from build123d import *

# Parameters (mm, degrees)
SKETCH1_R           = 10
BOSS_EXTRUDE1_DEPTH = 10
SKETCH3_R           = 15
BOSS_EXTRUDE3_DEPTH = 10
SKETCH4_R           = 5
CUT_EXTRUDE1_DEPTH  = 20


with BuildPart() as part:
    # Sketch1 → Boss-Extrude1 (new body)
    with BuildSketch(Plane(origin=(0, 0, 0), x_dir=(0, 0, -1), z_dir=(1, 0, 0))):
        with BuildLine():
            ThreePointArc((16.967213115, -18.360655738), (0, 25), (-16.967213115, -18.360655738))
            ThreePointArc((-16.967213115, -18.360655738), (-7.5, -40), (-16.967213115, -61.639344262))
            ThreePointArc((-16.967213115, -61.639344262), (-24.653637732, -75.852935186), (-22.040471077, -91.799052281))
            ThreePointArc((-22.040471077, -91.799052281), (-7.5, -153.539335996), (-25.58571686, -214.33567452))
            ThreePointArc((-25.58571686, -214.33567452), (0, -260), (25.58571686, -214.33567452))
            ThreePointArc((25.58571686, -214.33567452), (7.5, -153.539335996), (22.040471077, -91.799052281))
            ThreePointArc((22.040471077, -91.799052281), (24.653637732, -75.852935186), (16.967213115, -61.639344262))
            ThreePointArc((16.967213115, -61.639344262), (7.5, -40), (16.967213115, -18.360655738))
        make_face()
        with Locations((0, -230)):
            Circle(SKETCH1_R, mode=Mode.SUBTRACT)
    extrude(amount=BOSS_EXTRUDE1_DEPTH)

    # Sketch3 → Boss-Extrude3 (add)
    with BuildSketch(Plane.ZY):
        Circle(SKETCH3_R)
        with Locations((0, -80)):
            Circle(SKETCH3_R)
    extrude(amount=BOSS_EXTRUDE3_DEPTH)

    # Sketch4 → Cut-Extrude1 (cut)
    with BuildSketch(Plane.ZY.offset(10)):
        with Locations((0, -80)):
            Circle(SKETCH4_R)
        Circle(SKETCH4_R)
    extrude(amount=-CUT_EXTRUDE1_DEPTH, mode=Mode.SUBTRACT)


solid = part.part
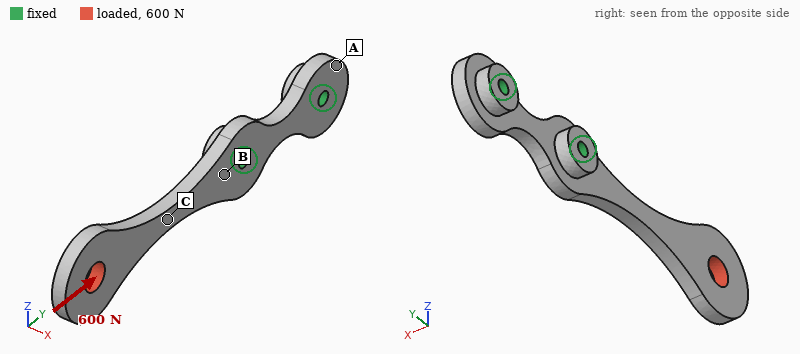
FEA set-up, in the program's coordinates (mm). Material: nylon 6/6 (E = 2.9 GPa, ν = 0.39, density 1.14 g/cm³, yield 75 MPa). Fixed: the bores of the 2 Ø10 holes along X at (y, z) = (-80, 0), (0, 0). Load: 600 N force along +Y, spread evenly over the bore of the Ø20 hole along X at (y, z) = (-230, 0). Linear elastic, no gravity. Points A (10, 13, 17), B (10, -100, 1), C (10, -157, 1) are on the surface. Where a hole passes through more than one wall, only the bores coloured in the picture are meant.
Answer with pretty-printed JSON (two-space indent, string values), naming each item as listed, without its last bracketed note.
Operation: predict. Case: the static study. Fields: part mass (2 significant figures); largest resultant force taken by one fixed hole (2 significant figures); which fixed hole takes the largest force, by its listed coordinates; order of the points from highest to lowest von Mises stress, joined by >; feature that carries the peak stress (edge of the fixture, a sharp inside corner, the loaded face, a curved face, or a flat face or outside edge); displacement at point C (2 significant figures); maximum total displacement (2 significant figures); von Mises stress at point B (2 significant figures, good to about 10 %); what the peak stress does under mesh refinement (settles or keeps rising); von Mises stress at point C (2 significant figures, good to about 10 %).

{
  "part mass": "120 g",
  "largest resultant force taken by one fixed hole": "580 N",
  "which fixed hole takes the largest force, by its listed coordinates": "(-80, 0)",
  "order of the points from highest to lowest von Mises stress, joined by >": "C > B > A",
  "feature that carries the peak stress": "edge of the fixture",
  "displacement at point C": "0.084 mm",
  "maximum total displacement": "0.17 mm",
  "von Mises stress at point B": "2.4 MPa",
  "what the peak stress does under mesh refinement": "keeps rising",
  "von Mises stress at point C": "3.8 MPa"
}
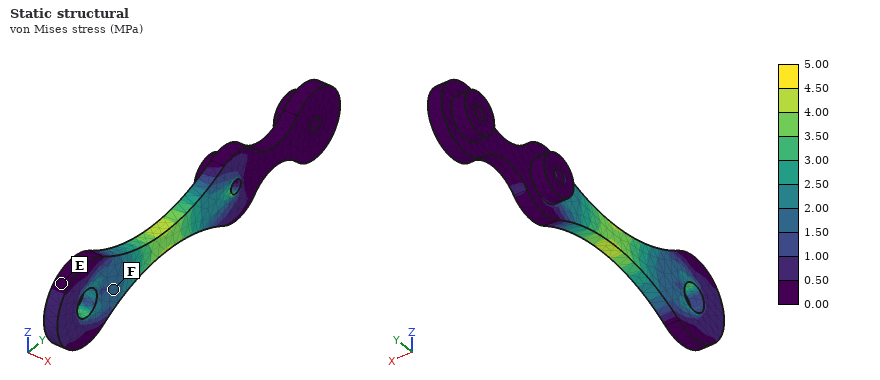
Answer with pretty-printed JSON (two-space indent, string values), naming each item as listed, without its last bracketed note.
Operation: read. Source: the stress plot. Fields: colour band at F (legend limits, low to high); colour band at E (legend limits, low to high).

{
  "colour band at F": "1.50 to 2.00 MPa",
  "colour band at E": "0.00 to 0.50 MPa"
}
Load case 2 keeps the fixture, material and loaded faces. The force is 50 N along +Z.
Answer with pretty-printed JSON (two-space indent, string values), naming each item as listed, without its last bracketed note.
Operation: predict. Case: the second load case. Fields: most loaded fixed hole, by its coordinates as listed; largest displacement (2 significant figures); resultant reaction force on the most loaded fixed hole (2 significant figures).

{
  "most loaded fixed hole, by its coordinates as listed": "(-80, 0)",
  "largest displacement": "3.2 mm",
  "resultant reaction force on the most loaded fixed hole": "89 N"
}
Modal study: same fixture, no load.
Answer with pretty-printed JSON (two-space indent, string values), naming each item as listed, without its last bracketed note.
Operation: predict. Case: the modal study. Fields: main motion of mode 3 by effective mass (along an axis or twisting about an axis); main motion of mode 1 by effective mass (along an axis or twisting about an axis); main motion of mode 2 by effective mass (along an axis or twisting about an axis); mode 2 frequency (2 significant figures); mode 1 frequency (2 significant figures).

{
  "main motion of mode 3 by effective mass": "twisting about Y",
  "main motion of mode 1 by effective mass": "along X",
  "main motion of mode 2 by effective mass": "along Z",
  "mode 2 frequency": "130 Hz",
  "mode 1 frequency": "67 Hz"
}
